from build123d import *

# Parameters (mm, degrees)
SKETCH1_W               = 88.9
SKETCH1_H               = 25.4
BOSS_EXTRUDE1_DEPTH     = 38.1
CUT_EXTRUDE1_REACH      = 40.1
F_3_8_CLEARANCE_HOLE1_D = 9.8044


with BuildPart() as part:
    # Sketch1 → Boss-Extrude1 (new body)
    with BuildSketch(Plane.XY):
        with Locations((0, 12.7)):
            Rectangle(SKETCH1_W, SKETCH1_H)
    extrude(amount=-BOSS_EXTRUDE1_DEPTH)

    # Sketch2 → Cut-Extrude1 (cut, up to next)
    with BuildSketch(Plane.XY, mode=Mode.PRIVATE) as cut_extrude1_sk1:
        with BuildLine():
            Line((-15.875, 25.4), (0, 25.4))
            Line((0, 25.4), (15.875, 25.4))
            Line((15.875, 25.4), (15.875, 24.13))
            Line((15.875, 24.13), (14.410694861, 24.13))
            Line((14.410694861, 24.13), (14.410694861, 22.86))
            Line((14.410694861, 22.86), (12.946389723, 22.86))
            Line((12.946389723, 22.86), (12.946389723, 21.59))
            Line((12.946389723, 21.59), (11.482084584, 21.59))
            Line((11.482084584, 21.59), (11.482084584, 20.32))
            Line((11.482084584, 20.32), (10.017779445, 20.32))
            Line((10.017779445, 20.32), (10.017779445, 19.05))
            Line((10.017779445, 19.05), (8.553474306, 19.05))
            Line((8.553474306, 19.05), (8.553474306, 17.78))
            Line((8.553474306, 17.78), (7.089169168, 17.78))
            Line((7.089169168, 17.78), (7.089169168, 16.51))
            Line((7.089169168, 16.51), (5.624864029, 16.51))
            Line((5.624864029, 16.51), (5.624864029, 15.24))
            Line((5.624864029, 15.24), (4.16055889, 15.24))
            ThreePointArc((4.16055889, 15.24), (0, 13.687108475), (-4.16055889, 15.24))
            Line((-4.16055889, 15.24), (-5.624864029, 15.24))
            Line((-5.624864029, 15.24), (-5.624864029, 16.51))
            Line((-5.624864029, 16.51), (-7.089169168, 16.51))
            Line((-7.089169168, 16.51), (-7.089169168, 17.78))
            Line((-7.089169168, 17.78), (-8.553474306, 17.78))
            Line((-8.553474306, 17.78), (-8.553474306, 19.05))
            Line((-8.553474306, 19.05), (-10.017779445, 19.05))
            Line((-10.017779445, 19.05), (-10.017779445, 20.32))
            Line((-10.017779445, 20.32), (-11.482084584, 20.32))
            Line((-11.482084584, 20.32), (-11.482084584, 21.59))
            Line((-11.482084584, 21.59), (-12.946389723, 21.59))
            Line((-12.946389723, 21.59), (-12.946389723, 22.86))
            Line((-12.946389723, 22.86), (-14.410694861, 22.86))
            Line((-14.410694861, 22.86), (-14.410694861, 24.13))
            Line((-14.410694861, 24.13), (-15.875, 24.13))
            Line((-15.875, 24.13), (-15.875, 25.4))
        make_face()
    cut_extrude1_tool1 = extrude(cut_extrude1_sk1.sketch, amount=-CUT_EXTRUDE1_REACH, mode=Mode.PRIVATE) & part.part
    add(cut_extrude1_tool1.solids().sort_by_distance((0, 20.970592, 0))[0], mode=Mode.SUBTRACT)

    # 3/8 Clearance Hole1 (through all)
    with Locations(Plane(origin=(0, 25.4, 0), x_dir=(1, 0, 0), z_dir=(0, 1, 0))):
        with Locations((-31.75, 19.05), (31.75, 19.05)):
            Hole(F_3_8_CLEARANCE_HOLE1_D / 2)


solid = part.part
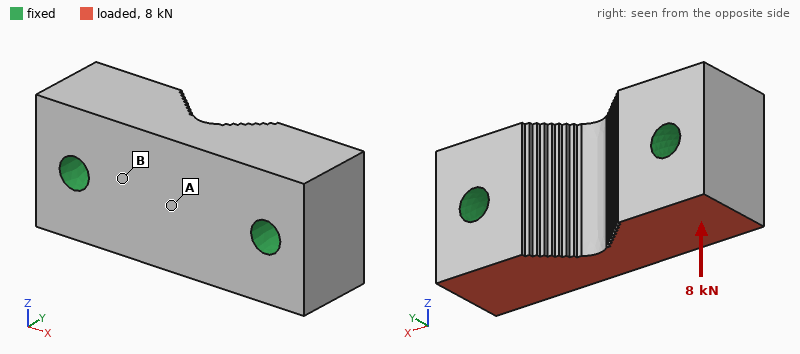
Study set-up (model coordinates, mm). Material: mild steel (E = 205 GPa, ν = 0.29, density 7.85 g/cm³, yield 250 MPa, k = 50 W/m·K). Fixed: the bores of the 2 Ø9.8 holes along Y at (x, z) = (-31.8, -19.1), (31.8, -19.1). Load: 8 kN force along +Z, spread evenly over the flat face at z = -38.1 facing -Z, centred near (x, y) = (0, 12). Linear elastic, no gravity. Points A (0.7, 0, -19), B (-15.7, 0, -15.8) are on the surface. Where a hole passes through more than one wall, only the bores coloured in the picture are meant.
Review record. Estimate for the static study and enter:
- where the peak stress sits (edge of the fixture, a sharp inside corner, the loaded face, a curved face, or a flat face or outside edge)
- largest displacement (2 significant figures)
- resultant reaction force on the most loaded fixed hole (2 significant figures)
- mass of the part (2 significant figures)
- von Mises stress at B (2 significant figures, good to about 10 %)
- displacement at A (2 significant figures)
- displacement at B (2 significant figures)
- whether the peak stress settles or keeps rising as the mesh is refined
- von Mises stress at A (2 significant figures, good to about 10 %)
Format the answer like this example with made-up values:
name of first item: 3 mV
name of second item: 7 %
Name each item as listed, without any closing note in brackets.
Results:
where the peak stress sits: edge of the fixture
largest displacement: 1.4 µm
resultant reaction force on the most loaded fixed hole: 4.0 kN
mass of the part: 580 g
von Mises stress at B: 4.7 MPa
displacement at A: 1.1 µm
displacement at B: 0.74 µm
whether the peak stress settles or keeps rising as the mesh is refined: keeps rising
von Mises stress at A: 1.8 MPa
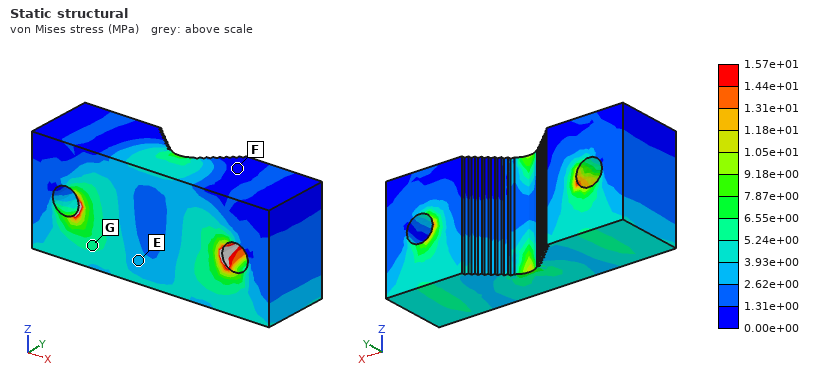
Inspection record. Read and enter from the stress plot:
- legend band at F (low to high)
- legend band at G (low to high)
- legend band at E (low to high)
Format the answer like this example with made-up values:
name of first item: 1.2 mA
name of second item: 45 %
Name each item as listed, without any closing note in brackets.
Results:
legend band at F: 0.00e+00 to 1.31e+00 MPa
legend band at G: 5.24e+00 to 6.55e+00 MPa
legend band at E: 2.62e+00 to 3.93e+00 MPa
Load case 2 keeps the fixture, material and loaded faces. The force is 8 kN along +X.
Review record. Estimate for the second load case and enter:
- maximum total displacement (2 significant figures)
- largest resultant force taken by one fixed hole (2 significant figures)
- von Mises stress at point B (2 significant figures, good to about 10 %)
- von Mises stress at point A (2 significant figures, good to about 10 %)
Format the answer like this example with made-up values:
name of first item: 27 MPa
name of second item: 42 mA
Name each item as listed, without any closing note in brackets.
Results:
maximum total displacement: 2.1 µm
largest resultant force taken by one fixed hole: 4.4 kN
von Mises stress at point B: 3.6 MPa
von Mises stress at point A: 4.5 MPa
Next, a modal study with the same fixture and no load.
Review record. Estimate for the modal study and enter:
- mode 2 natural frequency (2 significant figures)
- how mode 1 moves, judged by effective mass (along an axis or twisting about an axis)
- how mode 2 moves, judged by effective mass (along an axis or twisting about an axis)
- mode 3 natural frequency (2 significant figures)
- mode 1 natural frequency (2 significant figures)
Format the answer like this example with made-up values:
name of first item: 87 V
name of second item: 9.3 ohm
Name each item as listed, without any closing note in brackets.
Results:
mode 2 natural frequency: 19 kHz
how mode 1 moves, judged by effective mass: along Z
how mode 2 moves, judged by effective mass: along Y
mode 3 natural frequency: 24 kHz
mode 1 natural frequency: 18 kHz
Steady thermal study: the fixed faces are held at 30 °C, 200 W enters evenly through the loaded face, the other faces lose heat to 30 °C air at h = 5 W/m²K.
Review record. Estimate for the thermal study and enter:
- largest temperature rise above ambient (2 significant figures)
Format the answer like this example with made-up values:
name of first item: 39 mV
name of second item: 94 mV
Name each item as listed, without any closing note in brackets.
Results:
largest temperature rise above ambient: 52 K
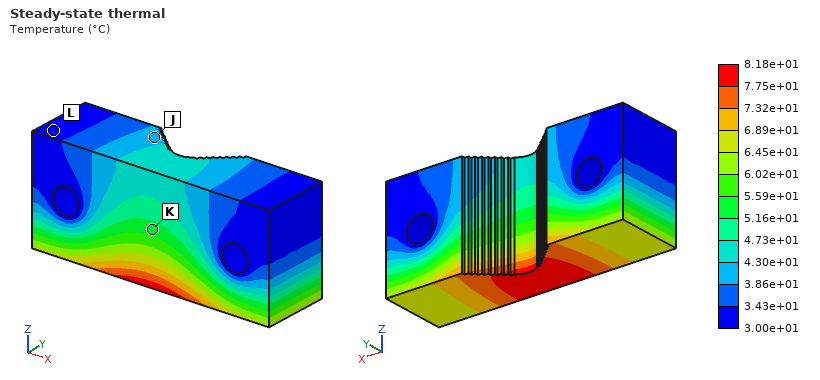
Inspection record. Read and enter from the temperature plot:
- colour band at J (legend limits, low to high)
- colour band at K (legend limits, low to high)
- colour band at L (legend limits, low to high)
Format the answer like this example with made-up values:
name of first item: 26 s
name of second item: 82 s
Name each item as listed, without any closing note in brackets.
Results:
colour band at J: 3.86e+01 to 4.30e+01 °C
colour band at K: 5.16e+01 to 5.59e+01 °C
colour band at L: 3.00e+01 to 3.43e+01 °C
